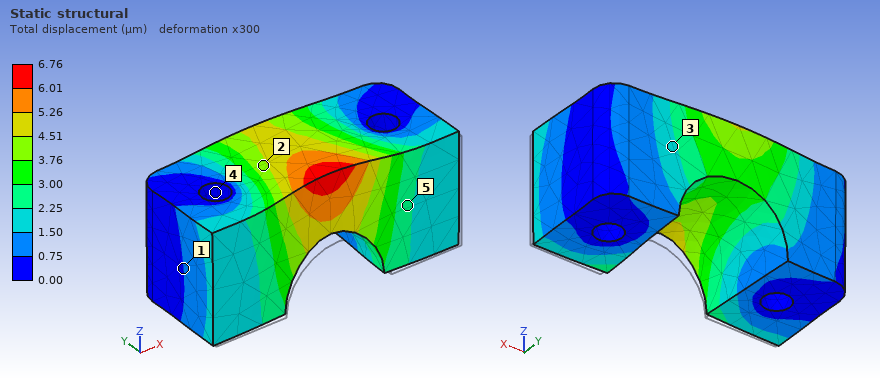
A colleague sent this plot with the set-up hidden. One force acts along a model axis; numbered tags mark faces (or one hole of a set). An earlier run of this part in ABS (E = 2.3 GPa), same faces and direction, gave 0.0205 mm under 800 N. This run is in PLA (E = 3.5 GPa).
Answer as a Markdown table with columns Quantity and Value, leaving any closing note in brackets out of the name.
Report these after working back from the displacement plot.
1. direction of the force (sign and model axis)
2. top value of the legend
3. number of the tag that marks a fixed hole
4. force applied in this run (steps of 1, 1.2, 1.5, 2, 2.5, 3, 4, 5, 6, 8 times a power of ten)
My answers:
| Quantity | Value |
|---|---|
| direction of the force | +Y |
| top value of the legend | 6.76 µm |
| number of the tag that marks a fixed hole | 4 |
| force applied in this run | 400 N |
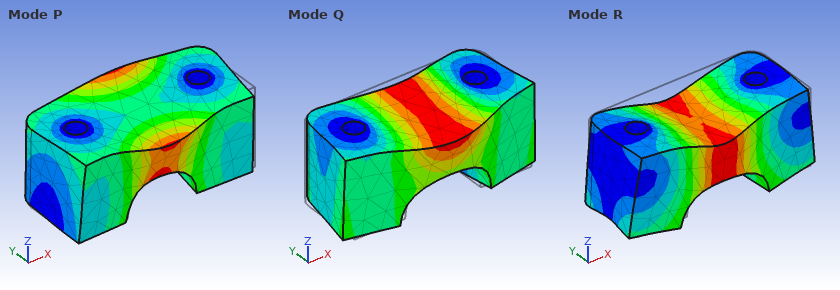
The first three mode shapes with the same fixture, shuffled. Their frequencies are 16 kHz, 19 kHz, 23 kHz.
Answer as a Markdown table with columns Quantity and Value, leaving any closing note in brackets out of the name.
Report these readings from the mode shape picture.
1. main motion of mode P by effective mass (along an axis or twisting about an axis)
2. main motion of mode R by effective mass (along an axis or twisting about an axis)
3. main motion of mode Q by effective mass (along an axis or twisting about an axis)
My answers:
| Quantity | Value |
|---|---|
| main motion of mode P by effective mass | twisting about X |
| main motion of mode R by effective mass | along Z |
| main motion of mode Q by effective mass | along Y |
